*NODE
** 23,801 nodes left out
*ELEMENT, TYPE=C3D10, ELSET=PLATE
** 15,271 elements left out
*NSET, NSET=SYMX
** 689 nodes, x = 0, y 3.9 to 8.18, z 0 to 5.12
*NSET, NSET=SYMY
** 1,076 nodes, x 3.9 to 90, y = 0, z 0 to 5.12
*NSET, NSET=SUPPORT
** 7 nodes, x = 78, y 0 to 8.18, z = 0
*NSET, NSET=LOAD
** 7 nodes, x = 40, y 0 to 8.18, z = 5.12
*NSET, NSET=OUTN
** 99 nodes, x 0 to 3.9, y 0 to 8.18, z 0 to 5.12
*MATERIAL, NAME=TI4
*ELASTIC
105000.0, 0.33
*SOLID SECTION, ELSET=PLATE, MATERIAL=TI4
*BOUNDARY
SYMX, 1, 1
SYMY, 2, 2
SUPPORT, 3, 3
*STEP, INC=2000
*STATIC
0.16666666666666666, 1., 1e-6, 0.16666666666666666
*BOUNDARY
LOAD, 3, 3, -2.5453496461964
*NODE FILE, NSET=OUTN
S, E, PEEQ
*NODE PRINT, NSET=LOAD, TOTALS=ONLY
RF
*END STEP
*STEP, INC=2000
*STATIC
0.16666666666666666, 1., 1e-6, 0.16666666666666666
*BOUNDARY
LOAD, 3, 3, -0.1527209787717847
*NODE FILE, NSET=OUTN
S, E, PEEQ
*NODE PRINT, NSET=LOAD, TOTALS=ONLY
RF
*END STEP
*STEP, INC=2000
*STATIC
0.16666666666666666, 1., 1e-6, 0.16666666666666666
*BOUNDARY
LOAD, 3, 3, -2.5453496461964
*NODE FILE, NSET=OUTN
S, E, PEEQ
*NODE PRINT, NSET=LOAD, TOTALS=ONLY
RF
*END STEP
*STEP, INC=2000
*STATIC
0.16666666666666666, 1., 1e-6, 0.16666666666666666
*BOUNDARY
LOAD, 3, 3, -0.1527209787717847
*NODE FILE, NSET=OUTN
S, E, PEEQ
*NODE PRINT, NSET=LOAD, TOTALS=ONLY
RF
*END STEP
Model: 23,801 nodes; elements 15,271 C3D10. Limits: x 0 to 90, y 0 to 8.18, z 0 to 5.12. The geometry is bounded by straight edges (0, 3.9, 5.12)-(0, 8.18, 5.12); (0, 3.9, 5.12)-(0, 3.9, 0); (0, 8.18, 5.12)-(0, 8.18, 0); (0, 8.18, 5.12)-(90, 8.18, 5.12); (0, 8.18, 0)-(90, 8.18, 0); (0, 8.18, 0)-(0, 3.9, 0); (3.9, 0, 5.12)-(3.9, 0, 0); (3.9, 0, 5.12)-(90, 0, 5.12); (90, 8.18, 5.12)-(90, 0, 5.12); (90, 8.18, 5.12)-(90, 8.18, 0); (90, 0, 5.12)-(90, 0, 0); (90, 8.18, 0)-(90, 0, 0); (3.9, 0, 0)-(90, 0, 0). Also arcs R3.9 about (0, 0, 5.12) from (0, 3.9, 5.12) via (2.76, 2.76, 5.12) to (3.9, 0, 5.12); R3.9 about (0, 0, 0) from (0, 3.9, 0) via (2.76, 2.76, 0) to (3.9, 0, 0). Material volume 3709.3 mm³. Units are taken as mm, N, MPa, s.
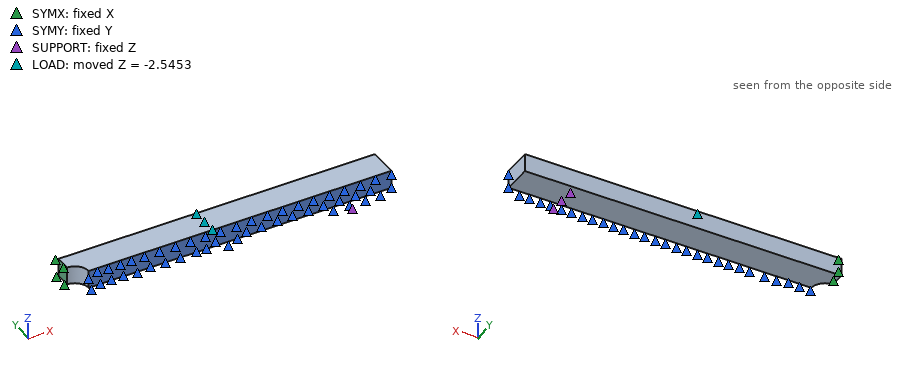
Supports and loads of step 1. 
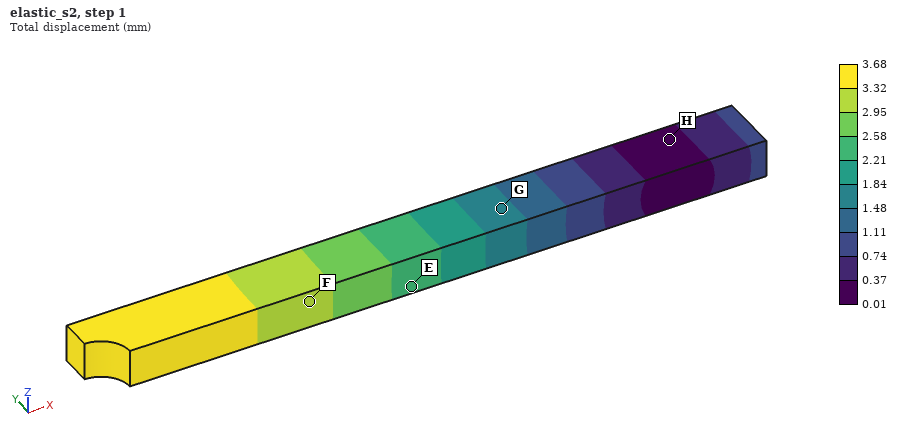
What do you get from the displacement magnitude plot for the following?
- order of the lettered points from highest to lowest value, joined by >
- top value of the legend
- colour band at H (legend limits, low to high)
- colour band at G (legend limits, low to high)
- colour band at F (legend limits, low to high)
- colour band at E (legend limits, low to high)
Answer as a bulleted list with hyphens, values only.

- F > E > G > H
- 3.68 mm
- 0.01 to 0.37 mm
- 1.48 to 1.84 mm
- 2.95 to 3.32 mm
- 2.21 to 2.58 mm
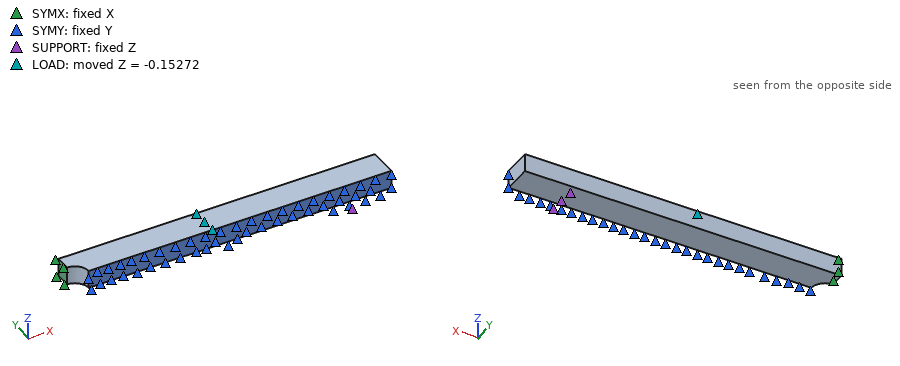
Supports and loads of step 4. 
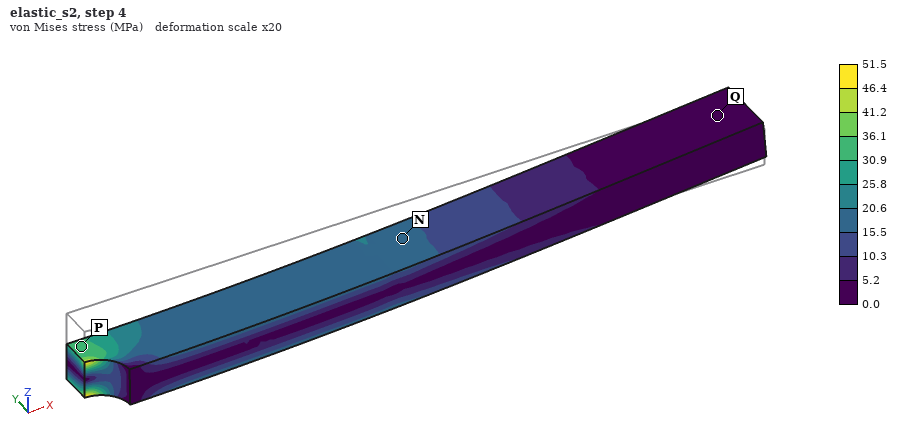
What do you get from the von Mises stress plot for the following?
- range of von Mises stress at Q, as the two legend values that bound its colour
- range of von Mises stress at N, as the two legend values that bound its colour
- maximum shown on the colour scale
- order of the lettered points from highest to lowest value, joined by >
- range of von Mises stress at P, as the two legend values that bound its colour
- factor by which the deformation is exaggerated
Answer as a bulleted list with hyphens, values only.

- 0.0 to 5.2 MPa
- 15.5 to 20.6 MPa
- 51.5 MPa
- P > N > Q
- 30.9 to 36.1 MPa
- 20
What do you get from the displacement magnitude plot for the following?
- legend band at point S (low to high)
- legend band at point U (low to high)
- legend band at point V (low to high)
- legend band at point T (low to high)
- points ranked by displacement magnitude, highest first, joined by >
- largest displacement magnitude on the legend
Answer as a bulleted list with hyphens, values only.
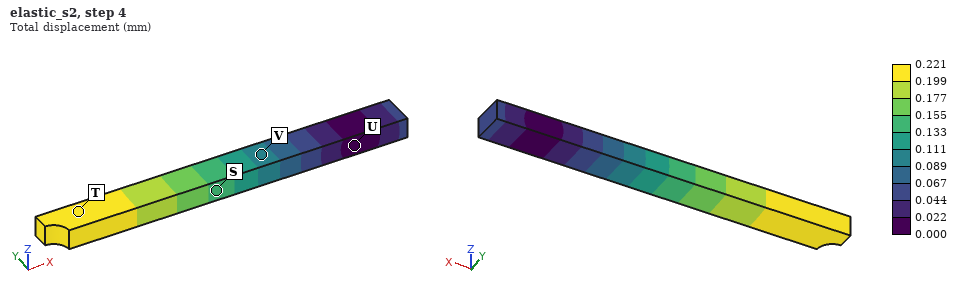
- 0.133 to 0.155 mm
- 0.000 to 0.022 mm
- 0.089 to 0.111 mm
- 0.199 to 0.221 mm
- T > S > V > U
- 0.221 mm
